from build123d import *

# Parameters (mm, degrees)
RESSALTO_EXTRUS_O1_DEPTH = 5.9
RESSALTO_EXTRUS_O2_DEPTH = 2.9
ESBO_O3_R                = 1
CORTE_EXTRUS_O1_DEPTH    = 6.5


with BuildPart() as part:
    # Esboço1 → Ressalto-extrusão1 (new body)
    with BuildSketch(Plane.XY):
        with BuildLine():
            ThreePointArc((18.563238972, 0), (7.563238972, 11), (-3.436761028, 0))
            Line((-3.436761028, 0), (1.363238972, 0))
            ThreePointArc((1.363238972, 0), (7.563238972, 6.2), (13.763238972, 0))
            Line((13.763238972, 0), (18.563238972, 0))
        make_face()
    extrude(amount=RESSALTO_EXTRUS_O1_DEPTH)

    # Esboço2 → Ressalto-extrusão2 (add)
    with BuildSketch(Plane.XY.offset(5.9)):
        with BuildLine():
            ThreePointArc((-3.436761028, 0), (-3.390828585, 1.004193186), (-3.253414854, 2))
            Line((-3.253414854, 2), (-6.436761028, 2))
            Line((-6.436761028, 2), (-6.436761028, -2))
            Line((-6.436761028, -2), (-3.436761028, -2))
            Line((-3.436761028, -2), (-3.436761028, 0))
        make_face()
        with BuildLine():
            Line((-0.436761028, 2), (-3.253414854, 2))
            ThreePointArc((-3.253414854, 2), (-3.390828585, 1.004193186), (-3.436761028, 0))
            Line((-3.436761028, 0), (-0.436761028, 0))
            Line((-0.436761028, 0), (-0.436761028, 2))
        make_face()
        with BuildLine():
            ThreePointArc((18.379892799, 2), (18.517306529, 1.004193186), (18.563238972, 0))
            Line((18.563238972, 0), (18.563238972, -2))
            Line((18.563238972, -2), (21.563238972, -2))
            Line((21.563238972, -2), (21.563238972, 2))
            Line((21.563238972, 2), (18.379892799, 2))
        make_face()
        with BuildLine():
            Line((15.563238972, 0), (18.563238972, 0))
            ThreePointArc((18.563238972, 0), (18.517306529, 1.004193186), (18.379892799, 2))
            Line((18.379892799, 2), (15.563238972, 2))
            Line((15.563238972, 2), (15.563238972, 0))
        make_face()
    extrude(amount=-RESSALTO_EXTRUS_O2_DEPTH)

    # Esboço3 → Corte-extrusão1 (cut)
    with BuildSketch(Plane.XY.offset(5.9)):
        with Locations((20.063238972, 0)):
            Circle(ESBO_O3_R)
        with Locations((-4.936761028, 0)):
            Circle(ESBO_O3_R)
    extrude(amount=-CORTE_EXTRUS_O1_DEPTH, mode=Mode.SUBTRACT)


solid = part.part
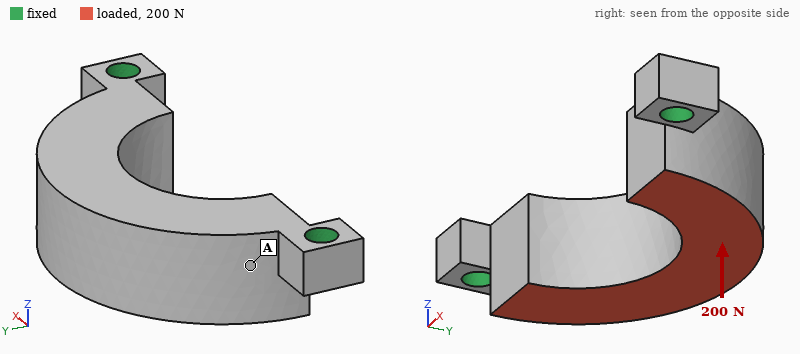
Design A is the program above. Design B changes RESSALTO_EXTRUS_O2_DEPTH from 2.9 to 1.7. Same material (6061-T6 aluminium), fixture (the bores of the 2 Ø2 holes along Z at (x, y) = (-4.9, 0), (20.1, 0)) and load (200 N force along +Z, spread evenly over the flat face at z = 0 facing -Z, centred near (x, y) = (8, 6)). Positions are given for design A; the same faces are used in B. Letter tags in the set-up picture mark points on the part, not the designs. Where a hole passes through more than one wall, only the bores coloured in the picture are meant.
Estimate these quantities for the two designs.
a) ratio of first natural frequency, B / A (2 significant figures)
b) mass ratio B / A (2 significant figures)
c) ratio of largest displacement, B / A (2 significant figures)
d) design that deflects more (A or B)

0.58
0.97
2.8
B
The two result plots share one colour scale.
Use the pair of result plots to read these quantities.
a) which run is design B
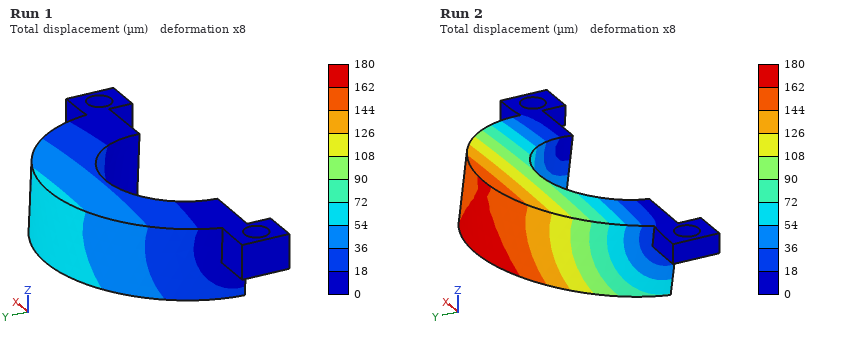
Run 2
